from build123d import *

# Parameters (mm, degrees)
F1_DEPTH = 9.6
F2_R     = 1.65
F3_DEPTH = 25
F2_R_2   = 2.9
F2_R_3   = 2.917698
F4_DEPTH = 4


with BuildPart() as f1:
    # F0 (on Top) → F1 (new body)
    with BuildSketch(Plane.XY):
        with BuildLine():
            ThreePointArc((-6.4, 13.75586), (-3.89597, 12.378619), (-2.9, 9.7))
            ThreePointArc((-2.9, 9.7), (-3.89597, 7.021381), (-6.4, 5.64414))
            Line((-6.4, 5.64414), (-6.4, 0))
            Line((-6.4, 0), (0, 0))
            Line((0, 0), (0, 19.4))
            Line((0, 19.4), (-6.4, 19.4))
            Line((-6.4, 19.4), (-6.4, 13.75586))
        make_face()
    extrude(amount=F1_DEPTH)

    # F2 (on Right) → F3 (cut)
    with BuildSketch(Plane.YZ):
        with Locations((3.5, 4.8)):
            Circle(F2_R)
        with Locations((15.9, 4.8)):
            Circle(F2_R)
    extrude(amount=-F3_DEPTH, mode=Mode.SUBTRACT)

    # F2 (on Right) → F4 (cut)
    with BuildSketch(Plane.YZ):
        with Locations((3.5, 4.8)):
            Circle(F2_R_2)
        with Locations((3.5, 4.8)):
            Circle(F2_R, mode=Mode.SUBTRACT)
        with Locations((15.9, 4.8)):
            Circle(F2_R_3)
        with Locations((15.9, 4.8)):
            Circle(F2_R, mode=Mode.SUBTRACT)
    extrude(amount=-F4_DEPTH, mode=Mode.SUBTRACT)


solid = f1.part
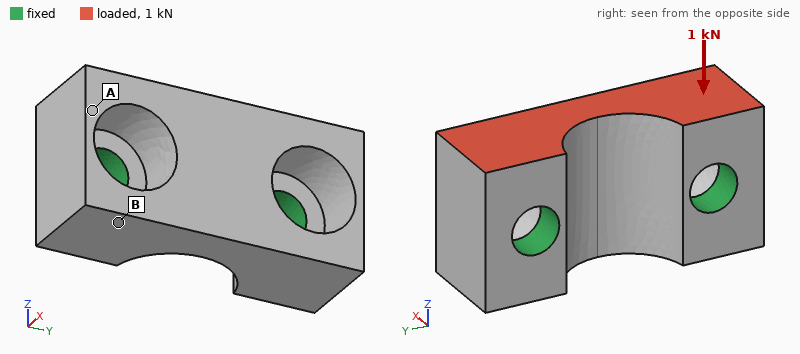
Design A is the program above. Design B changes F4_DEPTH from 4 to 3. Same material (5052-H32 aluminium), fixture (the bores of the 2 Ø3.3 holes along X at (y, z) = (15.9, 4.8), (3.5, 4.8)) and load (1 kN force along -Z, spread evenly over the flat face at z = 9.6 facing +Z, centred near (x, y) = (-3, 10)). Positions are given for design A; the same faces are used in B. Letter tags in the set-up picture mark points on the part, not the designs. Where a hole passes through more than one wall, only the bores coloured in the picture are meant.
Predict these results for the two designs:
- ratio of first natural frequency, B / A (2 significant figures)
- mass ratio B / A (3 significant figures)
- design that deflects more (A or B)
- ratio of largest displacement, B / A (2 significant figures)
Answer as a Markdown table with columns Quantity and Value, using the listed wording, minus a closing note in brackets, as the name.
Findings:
| Quantity | Value |
|---|---|
| ratio of first natural frequency, B / A | 1.4 |
| mass ratio B / A | 1.05 |
| design that deflects more | A |
| ratio of largest displacement, B / A | 0.51 |
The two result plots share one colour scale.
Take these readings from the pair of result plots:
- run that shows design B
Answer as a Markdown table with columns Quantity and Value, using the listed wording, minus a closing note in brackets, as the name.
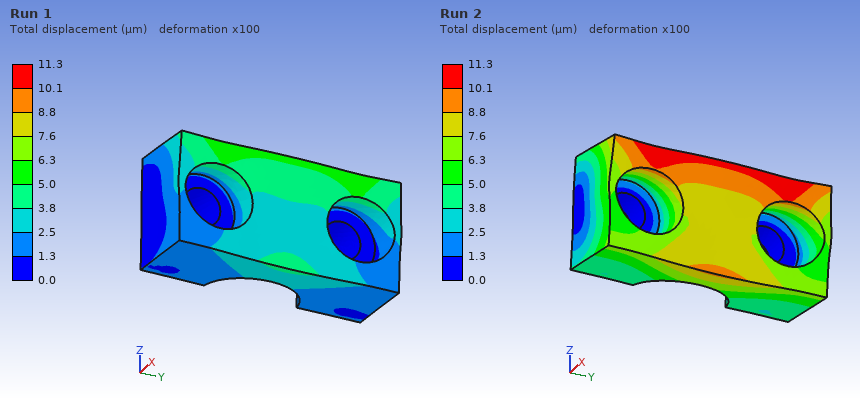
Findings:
| Quantity | Value |
|---|---|
| run that shows design B | Run 1 |
